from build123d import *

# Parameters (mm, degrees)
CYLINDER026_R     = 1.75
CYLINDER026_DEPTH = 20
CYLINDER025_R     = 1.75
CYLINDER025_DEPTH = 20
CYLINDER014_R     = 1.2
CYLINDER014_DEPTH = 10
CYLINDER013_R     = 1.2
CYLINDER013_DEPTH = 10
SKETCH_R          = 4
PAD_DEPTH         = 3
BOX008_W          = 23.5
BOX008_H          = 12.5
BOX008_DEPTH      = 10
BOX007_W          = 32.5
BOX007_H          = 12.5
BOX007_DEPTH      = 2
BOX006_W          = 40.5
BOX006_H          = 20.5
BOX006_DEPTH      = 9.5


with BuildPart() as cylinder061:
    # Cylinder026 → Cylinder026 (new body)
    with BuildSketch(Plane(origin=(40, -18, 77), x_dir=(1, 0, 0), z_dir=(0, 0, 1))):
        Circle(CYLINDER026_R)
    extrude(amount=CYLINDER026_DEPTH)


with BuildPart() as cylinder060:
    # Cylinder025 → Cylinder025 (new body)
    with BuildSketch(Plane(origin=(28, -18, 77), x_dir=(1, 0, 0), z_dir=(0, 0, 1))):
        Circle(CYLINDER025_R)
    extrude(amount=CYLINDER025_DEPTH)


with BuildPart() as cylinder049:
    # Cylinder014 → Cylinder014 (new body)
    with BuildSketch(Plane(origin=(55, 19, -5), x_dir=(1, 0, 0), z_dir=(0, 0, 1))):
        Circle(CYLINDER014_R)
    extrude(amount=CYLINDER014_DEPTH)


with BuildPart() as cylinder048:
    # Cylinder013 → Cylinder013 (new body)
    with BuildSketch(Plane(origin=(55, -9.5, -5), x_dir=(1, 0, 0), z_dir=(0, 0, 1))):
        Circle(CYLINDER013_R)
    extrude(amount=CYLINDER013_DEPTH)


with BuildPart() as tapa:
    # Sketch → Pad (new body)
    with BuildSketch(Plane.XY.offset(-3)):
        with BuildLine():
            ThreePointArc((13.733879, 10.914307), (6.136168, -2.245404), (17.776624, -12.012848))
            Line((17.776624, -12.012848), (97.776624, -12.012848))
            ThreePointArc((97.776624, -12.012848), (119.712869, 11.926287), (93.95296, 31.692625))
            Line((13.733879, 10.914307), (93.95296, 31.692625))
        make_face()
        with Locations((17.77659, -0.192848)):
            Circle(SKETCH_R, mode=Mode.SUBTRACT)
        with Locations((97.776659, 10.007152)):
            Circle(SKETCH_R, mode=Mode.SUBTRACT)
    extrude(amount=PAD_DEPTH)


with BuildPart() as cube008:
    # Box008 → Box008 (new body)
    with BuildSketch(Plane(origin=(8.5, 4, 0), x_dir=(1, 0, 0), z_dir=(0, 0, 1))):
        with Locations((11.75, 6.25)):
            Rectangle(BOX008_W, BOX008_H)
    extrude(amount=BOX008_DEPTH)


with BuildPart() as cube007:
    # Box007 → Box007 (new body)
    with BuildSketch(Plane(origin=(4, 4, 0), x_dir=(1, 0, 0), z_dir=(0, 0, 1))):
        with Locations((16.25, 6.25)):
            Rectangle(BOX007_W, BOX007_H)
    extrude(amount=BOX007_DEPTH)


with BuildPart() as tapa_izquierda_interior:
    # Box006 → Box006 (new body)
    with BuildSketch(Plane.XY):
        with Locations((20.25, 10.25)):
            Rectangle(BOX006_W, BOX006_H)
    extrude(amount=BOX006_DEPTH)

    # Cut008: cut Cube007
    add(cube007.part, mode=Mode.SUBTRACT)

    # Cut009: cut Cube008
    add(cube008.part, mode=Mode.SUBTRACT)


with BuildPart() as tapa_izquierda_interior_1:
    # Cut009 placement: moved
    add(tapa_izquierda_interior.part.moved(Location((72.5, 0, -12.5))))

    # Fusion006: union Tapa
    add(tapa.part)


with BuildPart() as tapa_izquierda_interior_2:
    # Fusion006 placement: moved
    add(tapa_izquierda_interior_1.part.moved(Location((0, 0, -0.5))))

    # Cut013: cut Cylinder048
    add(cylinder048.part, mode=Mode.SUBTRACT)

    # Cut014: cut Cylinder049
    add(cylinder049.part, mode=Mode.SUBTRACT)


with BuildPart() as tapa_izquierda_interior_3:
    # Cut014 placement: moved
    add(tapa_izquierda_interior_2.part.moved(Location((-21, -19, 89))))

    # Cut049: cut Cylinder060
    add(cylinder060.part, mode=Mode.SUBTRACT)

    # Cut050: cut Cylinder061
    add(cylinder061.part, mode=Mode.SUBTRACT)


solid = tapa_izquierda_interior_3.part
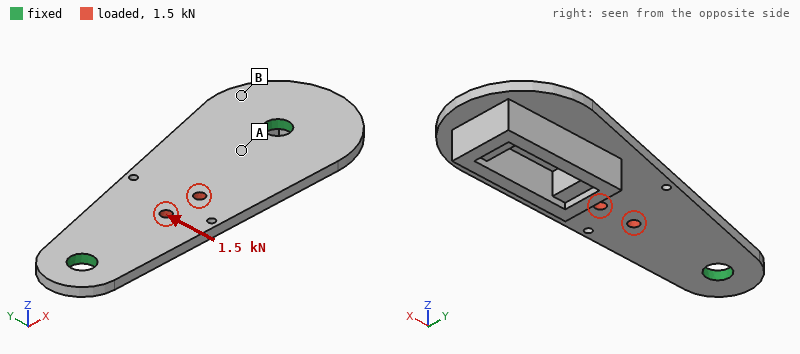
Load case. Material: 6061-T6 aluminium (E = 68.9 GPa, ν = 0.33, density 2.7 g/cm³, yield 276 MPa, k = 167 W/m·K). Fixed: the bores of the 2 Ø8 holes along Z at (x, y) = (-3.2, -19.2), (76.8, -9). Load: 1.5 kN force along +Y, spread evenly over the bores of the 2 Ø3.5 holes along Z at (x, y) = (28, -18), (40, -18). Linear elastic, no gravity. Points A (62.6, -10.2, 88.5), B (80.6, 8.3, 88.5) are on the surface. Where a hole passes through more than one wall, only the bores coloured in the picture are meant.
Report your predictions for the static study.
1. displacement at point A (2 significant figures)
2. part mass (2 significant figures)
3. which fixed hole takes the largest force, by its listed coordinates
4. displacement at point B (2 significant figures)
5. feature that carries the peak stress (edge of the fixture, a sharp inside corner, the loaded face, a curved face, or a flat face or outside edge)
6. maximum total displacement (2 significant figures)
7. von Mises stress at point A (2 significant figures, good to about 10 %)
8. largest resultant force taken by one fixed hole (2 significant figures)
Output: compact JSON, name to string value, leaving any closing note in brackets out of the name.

{"displacement at point A": "9.6 µm", "part mass": "42 g", "which fixed hole takes the largest force, by its listed coordinates": "(-3.2, -19.2)", "displacement at point B": "8.2 µm", "feature that carries the peak stress": "a curved face", "maximum total displacement": "27 µm", "von Mises stress at point A": "15 MPa", "largest resultant force taken by one fixed hole": "800 N"}
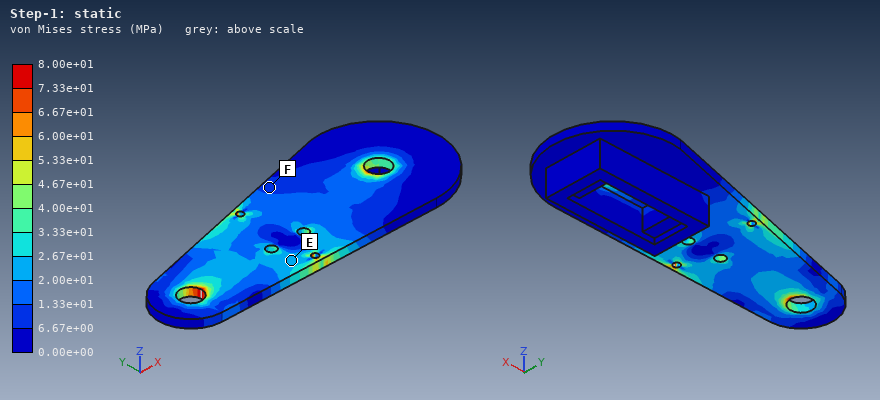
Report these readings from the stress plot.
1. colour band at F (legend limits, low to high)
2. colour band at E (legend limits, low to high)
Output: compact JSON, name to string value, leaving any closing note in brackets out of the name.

{"colour band at F": "6.67e+00 to 1.33e+01 MPa", "colour band at E": "2.00e+01 to 2.67e+01 MPa"}
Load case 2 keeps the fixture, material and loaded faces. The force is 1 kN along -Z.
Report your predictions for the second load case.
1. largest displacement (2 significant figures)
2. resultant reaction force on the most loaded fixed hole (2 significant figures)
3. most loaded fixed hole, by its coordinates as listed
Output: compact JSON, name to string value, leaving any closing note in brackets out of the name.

{"largest displacement": "0.33 mm", "resultant reaction force on the most loaded fixed hole": "640 N", "most loaded fixed hole, by its coordinates as listed": "(76.8, -9)"}
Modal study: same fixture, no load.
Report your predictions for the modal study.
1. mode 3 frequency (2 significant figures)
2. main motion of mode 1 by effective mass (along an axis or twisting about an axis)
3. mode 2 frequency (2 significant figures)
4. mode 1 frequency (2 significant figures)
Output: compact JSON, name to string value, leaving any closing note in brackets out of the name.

{"mode 3 frequency": "6500 Hz", "main motion of mode 1 by effective mass": "along Z", "mode 2 frequency": "4800 Hz", "mode 1 frequency": "3100 Hz"}
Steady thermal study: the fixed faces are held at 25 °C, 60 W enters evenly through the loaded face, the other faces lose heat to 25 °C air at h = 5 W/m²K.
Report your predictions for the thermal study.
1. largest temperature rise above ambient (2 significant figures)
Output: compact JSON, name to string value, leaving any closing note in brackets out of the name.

{"largest temperature rise above ambient": "73 K"}
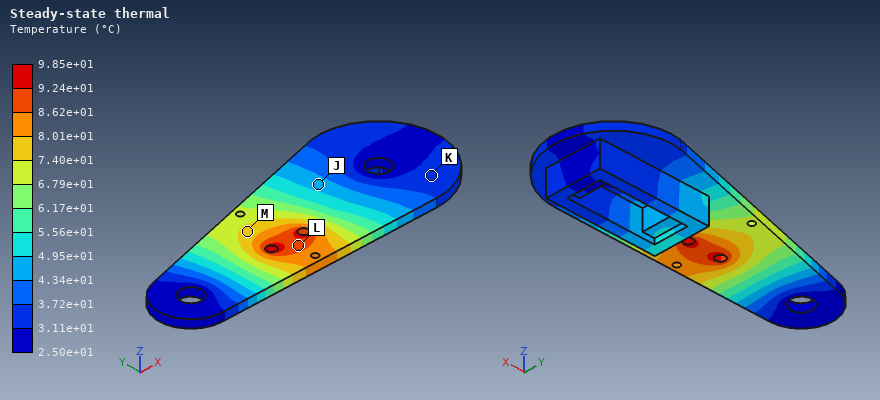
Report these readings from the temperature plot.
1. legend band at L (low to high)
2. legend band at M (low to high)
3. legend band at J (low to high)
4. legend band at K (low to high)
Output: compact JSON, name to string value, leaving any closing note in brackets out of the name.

{"legend band at L": "8.62e+01 to 9.24e+01 °C", "legend band at M": "7.40e+01 to 8.01e+01 °C", "legend band at J": "4.34e+01 to 4.95e+01 °C", "legend band at K": "3.11e+01 to 3.72e+01 °C"}
